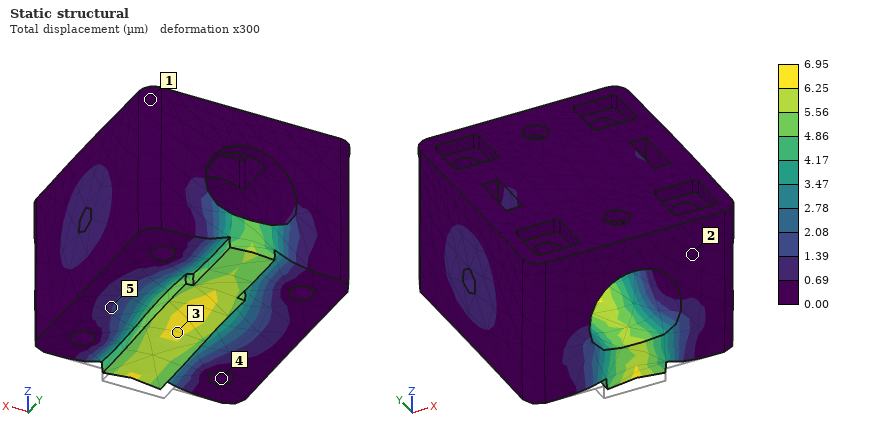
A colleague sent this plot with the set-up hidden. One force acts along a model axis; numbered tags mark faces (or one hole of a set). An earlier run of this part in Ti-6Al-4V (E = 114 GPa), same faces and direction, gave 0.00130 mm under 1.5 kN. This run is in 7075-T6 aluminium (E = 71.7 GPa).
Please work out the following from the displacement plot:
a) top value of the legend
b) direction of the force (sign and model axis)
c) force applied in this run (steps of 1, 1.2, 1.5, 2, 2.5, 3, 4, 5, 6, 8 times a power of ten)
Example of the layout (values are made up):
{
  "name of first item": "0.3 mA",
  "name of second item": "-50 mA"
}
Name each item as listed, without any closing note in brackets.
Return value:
{
  "top value of the legend": "6.95 µm",
  "direction of the force": "+Z",
  "force applied in this run": "5 kN"
}
